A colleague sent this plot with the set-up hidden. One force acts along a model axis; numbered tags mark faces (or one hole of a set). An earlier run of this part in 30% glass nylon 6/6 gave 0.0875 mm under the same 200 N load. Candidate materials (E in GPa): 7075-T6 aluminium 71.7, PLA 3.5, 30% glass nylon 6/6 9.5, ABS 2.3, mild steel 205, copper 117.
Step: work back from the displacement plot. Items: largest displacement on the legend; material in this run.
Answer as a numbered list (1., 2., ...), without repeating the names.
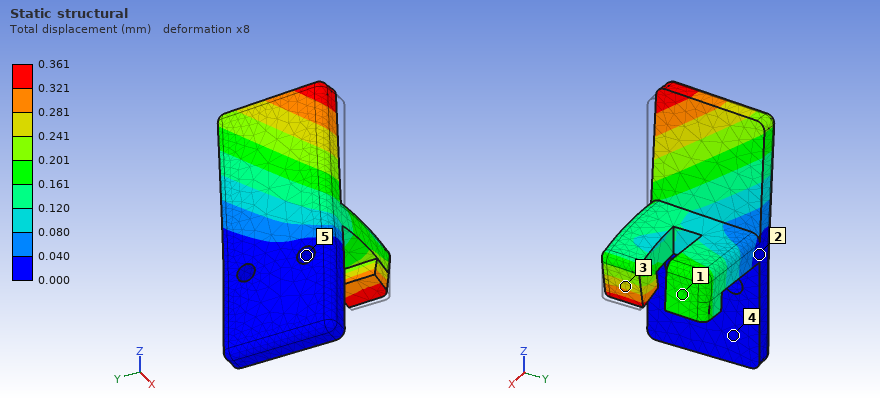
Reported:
1. 0.361 mm
2. ABS
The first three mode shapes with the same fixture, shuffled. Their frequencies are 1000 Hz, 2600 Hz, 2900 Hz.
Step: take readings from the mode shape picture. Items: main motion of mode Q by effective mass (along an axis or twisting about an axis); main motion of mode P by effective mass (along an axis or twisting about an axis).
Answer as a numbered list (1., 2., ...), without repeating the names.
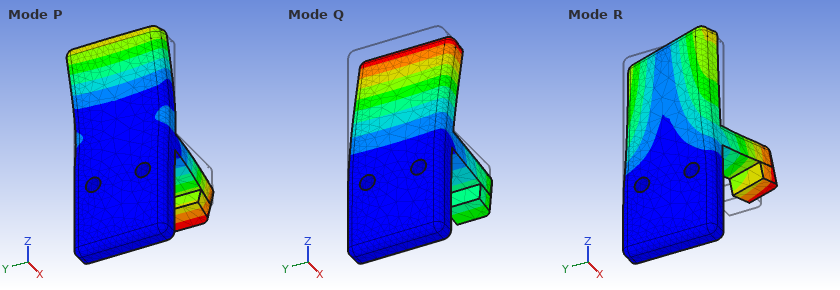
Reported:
1. along X
2. along Z
